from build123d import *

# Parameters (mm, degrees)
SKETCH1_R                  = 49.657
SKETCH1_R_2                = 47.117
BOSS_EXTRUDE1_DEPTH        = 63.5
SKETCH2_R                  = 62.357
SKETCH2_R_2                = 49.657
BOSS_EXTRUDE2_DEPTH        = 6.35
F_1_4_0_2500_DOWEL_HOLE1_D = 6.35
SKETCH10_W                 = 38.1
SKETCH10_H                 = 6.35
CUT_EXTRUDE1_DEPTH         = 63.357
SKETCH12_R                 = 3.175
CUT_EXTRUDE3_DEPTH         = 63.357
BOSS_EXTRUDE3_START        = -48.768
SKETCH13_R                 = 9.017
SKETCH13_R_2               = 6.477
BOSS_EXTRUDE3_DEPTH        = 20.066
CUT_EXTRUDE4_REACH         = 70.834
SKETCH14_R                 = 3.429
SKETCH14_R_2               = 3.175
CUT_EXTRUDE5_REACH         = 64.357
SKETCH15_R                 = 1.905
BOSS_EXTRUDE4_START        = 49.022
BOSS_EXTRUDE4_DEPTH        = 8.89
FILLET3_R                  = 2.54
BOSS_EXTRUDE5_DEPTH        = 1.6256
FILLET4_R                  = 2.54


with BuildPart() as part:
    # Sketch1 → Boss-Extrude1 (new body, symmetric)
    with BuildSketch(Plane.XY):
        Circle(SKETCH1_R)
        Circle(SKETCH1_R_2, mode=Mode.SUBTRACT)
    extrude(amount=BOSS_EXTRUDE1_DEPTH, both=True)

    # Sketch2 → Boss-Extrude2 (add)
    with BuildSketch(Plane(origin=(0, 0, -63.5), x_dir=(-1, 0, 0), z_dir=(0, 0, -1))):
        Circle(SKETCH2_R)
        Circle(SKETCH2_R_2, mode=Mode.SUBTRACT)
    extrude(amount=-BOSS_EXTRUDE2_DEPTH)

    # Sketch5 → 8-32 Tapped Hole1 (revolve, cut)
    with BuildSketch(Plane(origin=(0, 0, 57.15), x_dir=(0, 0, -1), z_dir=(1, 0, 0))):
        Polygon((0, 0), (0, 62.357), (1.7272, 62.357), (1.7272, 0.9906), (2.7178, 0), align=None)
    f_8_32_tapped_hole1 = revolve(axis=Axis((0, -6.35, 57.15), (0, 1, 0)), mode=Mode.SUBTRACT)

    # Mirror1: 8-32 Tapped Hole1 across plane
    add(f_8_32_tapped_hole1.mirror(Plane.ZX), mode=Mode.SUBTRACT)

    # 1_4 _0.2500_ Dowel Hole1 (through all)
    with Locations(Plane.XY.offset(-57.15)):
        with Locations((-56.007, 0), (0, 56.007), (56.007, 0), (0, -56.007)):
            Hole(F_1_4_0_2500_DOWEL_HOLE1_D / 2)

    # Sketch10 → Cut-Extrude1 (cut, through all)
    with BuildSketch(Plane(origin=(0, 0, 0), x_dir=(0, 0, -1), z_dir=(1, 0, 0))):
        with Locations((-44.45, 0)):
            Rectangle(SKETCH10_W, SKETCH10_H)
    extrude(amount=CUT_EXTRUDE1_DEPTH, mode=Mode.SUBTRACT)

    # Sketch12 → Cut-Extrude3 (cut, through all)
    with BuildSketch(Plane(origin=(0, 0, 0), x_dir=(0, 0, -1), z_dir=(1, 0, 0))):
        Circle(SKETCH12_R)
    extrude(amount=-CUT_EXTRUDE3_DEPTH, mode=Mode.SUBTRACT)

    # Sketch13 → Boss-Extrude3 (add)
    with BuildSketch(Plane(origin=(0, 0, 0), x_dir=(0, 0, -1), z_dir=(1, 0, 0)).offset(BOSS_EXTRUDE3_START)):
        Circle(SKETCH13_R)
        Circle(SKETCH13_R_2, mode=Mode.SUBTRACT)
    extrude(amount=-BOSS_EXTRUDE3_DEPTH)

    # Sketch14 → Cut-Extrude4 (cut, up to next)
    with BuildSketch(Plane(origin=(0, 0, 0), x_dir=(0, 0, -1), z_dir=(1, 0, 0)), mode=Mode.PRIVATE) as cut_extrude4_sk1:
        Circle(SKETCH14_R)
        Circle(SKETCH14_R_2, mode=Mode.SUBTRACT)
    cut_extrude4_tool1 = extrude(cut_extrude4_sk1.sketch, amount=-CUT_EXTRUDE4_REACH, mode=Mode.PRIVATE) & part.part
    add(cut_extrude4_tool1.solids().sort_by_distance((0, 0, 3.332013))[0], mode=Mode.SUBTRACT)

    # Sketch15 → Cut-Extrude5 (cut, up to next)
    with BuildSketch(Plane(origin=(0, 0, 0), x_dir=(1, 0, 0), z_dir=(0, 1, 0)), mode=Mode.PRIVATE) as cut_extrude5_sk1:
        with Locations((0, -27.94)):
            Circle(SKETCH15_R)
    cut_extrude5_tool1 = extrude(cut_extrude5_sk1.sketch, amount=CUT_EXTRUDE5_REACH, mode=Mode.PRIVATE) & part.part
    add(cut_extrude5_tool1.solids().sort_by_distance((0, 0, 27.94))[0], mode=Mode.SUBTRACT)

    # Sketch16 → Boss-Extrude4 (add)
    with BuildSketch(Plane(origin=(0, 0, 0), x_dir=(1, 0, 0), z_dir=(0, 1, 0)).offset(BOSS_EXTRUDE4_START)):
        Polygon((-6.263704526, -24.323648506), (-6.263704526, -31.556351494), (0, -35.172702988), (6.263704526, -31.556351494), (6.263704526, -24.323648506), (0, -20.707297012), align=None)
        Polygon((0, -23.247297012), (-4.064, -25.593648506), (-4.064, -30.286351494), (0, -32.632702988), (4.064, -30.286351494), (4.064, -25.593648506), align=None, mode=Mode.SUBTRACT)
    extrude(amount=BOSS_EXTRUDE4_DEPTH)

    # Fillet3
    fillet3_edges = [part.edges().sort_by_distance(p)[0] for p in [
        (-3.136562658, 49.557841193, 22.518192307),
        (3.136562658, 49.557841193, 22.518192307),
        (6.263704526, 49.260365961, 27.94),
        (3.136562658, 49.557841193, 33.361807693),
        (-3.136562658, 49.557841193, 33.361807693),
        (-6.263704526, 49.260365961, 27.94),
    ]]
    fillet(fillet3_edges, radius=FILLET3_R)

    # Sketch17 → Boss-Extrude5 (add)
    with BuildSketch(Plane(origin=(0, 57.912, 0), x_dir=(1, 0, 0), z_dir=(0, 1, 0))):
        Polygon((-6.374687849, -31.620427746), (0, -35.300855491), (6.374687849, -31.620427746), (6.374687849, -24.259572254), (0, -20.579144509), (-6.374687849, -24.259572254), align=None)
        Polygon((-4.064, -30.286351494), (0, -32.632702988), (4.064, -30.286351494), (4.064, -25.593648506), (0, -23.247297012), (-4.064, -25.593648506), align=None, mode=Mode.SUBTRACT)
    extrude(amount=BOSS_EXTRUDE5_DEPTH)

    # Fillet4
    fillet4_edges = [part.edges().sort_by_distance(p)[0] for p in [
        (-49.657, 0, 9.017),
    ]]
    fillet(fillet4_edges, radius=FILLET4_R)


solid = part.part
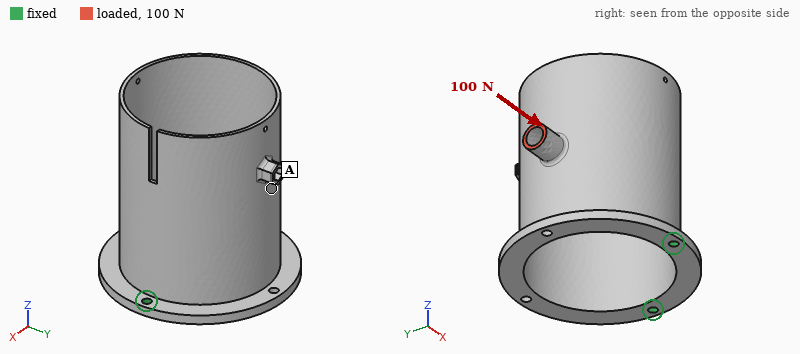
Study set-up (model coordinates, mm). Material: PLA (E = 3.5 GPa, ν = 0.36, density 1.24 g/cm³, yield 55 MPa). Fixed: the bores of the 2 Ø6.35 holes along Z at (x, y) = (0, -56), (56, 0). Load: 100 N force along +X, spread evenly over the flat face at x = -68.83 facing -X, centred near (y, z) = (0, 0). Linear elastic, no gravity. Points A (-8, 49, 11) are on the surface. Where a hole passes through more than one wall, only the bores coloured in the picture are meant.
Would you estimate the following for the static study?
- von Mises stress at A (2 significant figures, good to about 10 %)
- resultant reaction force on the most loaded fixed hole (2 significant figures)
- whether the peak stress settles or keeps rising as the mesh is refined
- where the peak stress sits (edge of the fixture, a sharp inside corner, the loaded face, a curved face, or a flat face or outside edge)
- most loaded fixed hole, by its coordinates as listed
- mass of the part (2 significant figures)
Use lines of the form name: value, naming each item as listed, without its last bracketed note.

von Mises stress at A: 1.7 MPa
resultant reaction force on the most loaded fixed hole: 85 N
whether the peak stress settles or keeps rising as the mesh is refined: keeps rising
where the peak stress sits: edge of the fixture
most loaded fixed hole, by its coordinates as listed: (56, 0)
mass of the part: 160 g
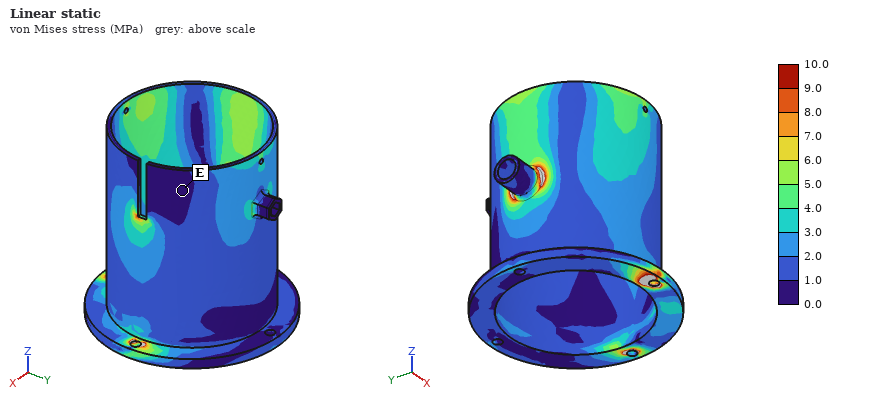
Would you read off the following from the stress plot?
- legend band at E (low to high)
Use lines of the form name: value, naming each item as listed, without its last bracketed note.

legend band at E: 0.0 to 1.0 MPa
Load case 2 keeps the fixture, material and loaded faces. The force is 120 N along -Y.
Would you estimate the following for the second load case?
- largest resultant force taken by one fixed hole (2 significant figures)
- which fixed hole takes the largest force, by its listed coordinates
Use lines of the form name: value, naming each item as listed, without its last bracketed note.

largest resultant force taken by one fixed hole: 170 N
which fixed hole takes the largest force, by its listed coordinates: (0, -56)
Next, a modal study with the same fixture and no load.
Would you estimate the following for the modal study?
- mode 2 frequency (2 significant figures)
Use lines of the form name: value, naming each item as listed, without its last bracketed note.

mode 2 frequency: 210 Hz
